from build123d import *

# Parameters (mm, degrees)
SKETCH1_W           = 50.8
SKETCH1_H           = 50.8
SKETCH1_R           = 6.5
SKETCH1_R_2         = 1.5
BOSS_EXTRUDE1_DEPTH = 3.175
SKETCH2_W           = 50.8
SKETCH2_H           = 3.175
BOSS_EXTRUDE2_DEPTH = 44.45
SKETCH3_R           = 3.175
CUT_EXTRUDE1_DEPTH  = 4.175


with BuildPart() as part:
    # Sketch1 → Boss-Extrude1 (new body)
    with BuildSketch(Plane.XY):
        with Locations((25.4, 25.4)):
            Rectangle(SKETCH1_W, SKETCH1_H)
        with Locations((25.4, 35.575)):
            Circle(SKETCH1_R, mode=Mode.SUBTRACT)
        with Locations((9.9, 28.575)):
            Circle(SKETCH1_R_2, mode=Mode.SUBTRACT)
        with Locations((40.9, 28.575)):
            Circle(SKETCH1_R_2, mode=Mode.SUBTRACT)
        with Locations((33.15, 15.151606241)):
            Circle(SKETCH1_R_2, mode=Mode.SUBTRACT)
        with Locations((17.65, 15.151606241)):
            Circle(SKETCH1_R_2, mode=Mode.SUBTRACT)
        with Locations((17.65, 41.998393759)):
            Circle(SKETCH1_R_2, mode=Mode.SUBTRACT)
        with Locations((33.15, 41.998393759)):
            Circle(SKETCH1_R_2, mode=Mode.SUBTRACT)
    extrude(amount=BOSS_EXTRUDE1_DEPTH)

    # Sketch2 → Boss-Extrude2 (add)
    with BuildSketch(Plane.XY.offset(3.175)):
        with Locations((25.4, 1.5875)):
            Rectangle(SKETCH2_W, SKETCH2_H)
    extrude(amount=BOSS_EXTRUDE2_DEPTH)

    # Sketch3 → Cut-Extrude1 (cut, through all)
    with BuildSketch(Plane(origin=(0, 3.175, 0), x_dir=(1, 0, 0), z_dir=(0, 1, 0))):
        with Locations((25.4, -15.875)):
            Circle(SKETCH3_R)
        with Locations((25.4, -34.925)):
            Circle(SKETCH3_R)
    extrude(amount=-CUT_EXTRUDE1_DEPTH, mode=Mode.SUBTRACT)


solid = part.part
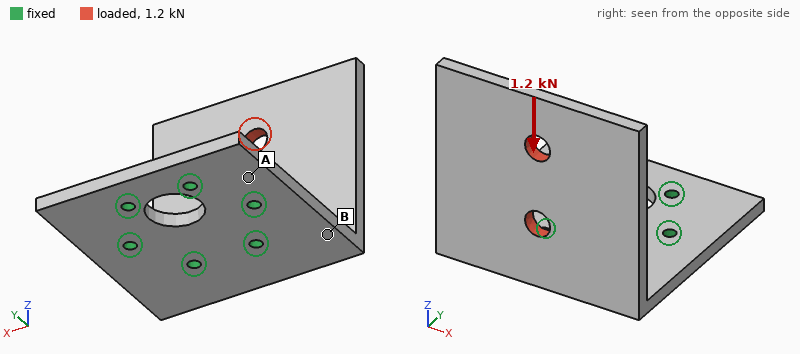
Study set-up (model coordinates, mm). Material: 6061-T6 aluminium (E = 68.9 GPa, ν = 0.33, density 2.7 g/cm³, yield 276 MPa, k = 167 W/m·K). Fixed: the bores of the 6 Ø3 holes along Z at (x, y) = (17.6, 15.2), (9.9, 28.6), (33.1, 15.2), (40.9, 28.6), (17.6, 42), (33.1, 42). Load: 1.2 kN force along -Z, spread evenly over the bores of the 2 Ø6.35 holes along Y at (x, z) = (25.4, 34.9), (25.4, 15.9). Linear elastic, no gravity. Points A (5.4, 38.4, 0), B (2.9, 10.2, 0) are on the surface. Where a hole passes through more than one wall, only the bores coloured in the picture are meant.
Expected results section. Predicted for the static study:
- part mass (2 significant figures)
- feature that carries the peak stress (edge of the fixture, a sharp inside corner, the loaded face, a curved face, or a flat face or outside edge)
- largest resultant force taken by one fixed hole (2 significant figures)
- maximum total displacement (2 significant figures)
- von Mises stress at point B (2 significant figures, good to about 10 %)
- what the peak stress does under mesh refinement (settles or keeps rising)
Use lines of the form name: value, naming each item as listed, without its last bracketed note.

part mass: 39 g
feature that carries the peak stress: edge of the fixture
largest resultant force taken by one fixed hole: 800 N
maximum total displacement: 0.62 mm
von Mises stress at point B: 71 MPa
what the peak stress does under mesh refinement: keeps rising
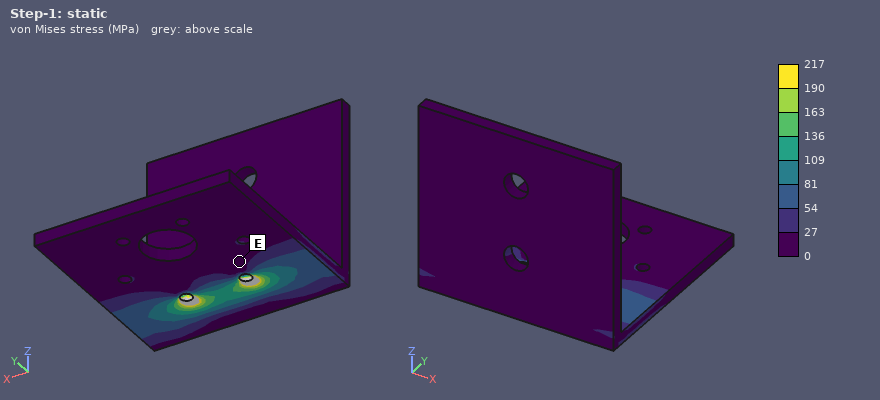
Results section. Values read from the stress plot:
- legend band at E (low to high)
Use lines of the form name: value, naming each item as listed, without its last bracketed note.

legend band at E: 0 to 27 MPa
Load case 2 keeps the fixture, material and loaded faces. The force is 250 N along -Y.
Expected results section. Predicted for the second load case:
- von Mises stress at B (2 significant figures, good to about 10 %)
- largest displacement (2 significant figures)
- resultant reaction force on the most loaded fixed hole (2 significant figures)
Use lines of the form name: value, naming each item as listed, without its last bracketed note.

von Mises stress at B: 54 MPa
largest displacement: 0.69 mm
resultant reaction force on the most loaded fixed hole: 150 N
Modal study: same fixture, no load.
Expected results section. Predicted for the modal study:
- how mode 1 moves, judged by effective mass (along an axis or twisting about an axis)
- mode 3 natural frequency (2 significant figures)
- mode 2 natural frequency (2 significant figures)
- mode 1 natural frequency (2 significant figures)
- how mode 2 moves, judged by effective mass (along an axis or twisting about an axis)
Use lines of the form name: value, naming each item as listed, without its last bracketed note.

how mode 1 moves, judged by effective mass: along Y
mode 3 natural frequency: 2700 Hz
mode 2 natural frequency: 1700 Hz
mode 1 natural frequency: 850 Hz
how mode 2 moves, judged by effective mass: along X
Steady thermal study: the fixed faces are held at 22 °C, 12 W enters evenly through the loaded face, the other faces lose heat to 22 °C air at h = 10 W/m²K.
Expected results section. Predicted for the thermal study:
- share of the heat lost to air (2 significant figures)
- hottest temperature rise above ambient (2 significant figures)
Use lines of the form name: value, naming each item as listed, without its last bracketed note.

share of the heat lost to air: 6.4 %
hottest temperature rise above ambient: 20 K
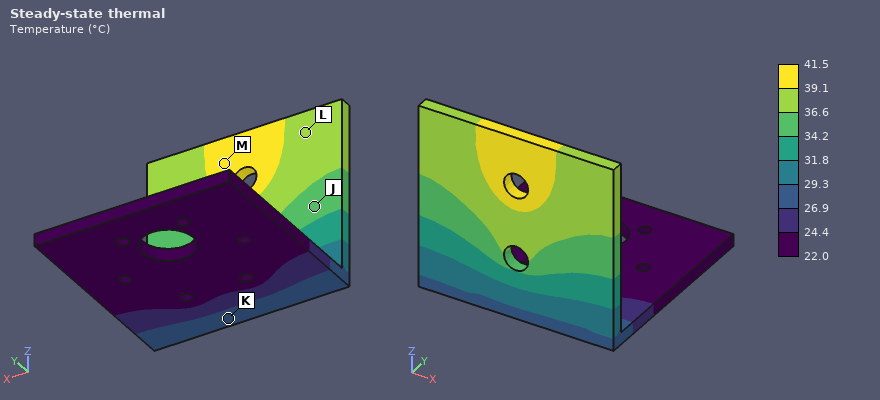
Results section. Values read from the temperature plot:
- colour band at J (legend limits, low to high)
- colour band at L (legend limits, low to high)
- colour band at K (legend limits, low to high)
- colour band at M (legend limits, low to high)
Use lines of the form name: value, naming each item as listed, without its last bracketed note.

colour band at J: 34.2 to 36.6 °C
colour band at L: 36.6 to 39.1 °C
colour band at K: 26.9 to 29.3 °C
colour band at M: 39.1 to 41.5 °C
